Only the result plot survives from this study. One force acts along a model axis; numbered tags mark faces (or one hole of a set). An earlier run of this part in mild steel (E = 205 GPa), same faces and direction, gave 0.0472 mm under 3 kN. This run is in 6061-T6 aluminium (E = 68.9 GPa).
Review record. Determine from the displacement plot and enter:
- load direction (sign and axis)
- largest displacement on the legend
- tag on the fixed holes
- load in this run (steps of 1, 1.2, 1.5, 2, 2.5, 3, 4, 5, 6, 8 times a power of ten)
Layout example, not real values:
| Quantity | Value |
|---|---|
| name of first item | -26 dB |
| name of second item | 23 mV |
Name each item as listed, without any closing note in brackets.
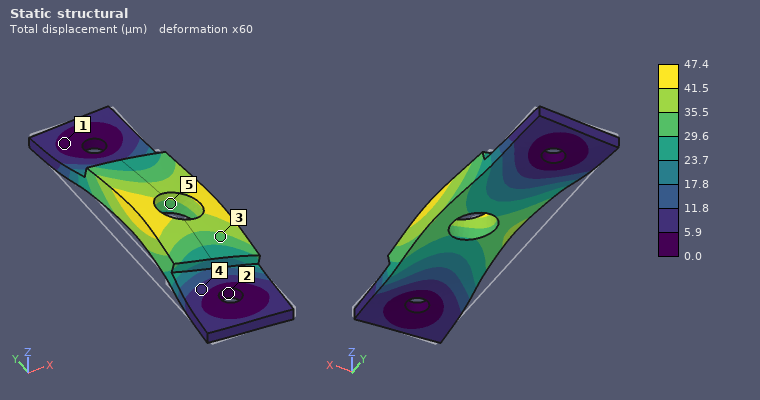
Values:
| Quantity | Value |
|---|---|
| load direction | +X |
| largest displacement on the legend | 47.4 µm |
| tag on the fixed holes | 2 |
| load in this run | 1 kN |
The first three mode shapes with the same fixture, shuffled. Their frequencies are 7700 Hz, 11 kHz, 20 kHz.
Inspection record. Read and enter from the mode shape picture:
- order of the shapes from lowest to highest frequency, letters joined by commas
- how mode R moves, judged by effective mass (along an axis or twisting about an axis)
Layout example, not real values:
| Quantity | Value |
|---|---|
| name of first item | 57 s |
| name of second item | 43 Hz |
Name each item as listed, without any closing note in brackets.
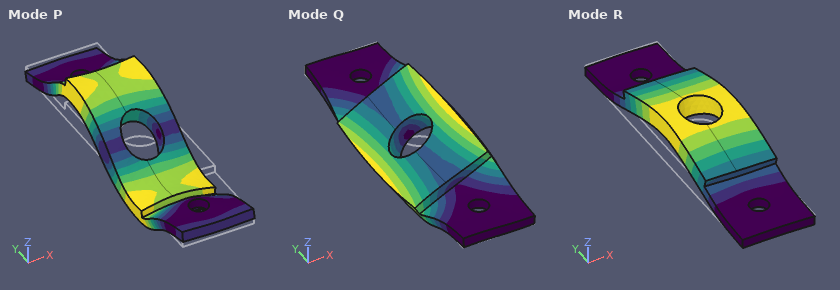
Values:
| Quantity | Value |
|---|---|
| order of the shapes from lowest to highest frequency, letters joined by commas | R, Q, P |
| how mode R moves, judged by effective mass | along Z |
